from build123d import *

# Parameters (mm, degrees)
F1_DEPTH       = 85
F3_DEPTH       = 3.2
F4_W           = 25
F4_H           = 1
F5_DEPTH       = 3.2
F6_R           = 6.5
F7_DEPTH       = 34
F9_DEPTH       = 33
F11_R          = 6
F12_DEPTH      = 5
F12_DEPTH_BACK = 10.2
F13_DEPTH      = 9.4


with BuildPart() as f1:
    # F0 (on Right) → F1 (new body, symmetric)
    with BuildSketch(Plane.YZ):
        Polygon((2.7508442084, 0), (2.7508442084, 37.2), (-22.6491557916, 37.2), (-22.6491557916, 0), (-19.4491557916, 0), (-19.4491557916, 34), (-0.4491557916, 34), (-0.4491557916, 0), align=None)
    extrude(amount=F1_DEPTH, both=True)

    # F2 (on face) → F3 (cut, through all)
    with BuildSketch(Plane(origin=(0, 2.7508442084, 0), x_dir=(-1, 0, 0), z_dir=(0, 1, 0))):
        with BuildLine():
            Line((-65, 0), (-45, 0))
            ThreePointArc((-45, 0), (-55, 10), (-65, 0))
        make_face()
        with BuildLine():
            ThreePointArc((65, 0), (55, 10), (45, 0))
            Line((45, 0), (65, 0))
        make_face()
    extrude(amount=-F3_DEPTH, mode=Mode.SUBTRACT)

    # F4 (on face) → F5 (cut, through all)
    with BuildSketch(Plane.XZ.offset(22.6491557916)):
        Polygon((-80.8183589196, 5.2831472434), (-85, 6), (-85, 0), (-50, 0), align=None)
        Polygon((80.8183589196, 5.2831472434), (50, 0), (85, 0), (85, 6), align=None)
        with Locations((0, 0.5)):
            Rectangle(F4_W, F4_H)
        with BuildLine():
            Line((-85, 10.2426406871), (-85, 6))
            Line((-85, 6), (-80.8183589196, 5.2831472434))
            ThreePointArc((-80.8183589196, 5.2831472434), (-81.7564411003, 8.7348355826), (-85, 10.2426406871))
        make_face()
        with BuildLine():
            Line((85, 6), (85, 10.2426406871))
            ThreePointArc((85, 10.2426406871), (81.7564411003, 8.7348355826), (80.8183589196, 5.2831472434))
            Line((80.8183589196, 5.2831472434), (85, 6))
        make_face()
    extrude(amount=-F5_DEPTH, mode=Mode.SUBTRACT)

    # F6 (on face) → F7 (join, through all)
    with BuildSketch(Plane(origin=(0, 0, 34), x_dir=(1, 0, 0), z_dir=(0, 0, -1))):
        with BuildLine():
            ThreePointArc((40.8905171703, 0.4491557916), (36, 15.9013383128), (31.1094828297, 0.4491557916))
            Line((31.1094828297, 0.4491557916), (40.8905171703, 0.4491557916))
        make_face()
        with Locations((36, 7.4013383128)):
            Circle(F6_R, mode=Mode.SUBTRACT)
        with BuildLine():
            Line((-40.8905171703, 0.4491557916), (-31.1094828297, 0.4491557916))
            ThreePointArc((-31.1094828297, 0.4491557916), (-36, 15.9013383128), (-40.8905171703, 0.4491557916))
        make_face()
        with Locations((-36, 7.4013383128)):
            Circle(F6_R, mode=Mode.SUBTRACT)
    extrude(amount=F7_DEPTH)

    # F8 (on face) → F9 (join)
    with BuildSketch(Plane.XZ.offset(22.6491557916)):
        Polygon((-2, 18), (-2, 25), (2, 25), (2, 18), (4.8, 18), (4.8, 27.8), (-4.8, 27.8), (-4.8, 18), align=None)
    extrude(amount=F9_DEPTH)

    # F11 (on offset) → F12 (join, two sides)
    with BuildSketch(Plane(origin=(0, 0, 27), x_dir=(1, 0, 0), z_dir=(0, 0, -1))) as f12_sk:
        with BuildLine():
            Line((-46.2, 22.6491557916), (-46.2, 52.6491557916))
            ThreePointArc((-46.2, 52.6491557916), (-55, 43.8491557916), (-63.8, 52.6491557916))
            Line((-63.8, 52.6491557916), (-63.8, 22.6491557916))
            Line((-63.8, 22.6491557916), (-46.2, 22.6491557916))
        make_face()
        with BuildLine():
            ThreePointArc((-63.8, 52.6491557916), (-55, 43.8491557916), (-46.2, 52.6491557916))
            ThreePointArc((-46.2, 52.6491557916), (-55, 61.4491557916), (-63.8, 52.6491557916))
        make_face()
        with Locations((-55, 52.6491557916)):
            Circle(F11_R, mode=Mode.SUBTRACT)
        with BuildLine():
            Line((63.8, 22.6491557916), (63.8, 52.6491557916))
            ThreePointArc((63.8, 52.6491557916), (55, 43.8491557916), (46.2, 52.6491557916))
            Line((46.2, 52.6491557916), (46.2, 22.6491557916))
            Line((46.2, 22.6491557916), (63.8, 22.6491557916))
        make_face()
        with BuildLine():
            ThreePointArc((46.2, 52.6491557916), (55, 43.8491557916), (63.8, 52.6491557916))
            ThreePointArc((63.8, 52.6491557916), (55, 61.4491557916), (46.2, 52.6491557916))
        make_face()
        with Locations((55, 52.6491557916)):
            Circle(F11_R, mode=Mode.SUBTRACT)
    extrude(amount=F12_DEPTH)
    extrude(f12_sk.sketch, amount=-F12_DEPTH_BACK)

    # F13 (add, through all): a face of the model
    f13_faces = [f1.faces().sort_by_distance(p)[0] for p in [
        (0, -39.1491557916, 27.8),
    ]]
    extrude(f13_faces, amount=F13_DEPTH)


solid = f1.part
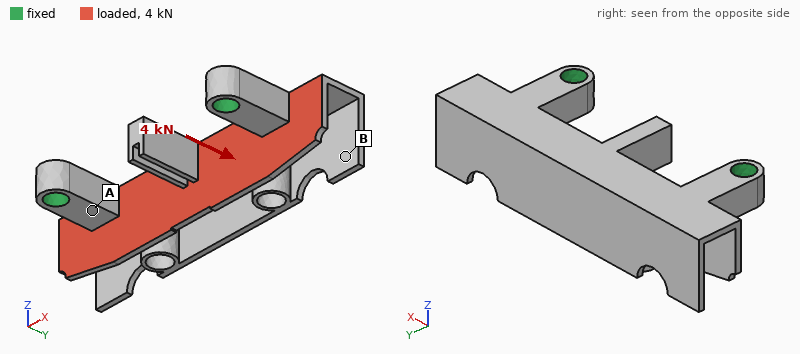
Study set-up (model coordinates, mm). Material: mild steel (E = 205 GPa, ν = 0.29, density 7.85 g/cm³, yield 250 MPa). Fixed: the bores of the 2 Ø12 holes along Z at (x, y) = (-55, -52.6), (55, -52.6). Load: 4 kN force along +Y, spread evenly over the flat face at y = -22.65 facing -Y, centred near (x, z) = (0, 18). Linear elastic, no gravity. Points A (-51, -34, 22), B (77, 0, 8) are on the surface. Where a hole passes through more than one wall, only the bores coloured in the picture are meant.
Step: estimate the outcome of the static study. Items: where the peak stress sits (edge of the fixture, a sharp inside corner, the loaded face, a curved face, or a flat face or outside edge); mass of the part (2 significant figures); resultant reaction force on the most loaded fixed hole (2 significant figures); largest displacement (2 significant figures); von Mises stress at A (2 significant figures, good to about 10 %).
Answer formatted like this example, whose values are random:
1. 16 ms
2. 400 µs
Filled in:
1. a flat face or outside edge
2. 600 g
3. 2.1 kN
4. 0.24 mm
5. 43 MPa
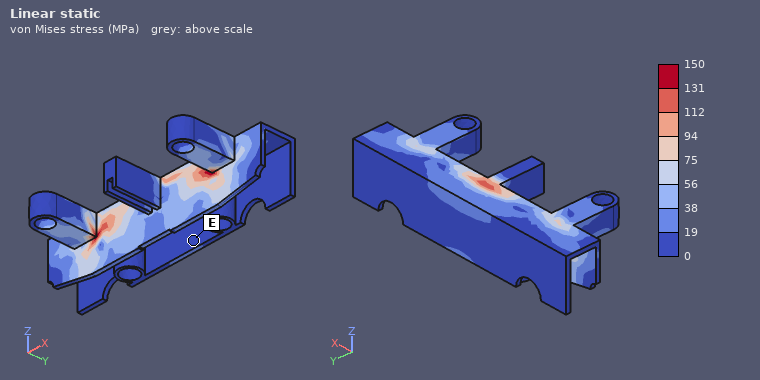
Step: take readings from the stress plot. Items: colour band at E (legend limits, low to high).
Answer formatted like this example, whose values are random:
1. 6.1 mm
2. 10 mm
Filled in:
1. 0 to 19 MPa
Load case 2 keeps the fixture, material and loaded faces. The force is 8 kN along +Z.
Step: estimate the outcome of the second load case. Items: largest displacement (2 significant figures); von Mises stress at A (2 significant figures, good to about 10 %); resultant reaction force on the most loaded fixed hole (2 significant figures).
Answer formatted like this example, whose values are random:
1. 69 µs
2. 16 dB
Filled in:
1. 57 µm
2. 75 MPa
3. 4.0 kN
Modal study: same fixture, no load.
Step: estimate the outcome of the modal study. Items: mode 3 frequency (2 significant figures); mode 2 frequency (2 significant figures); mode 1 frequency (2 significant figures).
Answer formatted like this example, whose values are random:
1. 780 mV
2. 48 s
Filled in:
1. 1900 Hz
2. 1500 Hz
3. 980 Hz
